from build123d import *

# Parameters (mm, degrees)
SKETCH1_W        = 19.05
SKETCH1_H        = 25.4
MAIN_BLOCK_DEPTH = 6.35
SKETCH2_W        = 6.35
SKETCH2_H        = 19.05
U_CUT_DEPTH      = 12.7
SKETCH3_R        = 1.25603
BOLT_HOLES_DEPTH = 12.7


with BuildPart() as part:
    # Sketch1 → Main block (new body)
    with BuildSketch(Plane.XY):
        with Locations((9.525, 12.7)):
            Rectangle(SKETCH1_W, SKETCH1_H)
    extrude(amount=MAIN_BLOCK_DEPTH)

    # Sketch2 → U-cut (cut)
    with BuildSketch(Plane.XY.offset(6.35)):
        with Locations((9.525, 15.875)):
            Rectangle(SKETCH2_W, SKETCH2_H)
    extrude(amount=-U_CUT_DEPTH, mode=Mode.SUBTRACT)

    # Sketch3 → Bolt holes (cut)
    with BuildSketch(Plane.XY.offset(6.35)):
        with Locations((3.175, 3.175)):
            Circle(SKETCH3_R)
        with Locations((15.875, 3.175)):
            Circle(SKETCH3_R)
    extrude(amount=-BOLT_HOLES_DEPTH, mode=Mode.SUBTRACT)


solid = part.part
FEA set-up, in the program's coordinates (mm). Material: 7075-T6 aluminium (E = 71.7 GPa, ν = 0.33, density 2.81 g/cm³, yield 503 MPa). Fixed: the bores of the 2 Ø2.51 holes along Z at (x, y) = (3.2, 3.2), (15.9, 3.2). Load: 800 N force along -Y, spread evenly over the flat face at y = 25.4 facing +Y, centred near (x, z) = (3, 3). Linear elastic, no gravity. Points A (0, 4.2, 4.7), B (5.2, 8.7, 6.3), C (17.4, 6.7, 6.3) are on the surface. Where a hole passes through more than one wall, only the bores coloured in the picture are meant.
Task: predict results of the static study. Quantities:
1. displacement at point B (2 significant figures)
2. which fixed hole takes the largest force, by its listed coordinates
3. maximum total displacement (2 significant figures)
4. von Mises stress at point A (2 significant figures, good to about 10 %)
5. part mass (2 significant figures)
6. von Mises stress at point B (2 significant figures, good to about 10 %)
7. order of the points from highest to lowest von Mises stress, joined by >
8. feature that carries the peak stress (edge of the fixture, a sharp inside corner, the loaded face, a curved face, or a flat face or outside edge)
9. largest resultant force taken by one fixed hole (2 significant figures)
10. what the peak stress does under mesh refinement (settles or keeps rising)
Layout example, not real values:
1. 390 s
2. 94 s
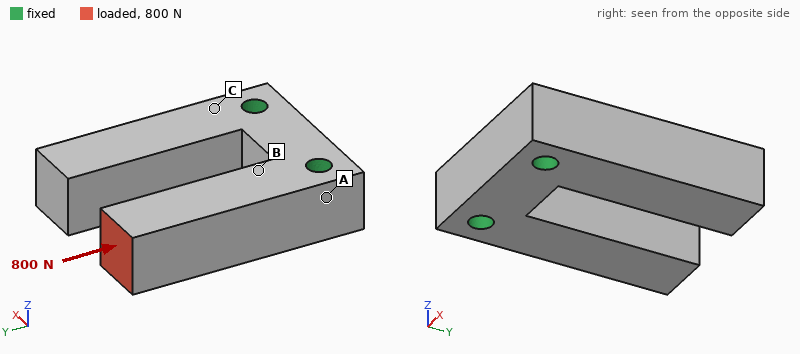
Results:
1. 1.4 µm
2. (3.2, 3.2)
3. 6.7 µm
4. 11 MPa
5. 6.3 g
6. 19 MPa
7. B > A > C
8. edge of the fixture
9. 780 N
10. keeps rising
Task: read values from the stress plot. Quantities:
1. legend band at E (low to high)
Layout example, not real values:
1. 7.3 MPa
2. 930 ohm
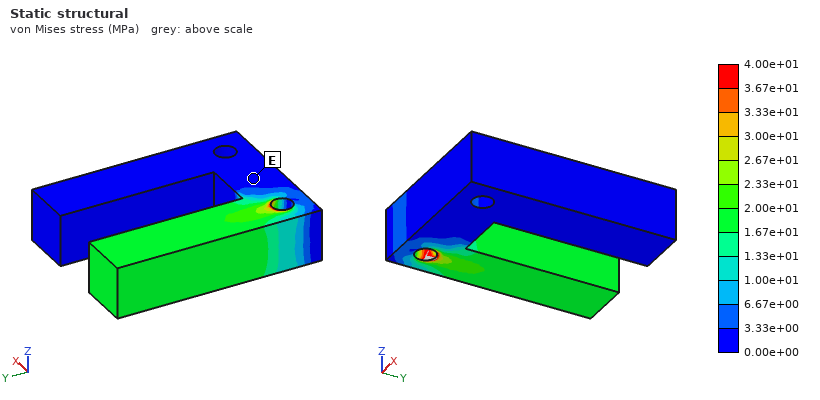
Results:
1. 0.00e+00 to 3.33e+00 MPa
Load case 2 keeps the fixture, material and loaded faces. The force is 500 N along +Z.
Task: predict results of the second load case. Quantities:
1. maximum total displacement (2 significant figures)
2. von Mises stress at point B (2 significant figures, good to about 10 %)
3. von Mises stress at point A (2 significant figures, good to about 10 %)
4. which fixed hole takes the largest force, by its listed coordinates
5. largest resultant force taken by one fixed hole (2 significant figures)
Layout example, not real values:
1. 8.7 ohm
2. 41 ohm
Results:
1. 0.19 mm
2. 200 MPa
3. 77 MPa
4. (3.2, 3.2)
5. 540 N
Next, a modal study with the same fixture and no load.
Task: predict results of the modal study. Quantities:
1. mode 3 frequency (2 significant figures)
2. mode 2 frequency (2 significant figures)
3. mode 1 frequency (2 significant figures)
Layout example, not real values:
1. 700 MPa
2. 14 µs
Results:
1. 10 kHz
2. 10 kHz
3. 9700 Hz
